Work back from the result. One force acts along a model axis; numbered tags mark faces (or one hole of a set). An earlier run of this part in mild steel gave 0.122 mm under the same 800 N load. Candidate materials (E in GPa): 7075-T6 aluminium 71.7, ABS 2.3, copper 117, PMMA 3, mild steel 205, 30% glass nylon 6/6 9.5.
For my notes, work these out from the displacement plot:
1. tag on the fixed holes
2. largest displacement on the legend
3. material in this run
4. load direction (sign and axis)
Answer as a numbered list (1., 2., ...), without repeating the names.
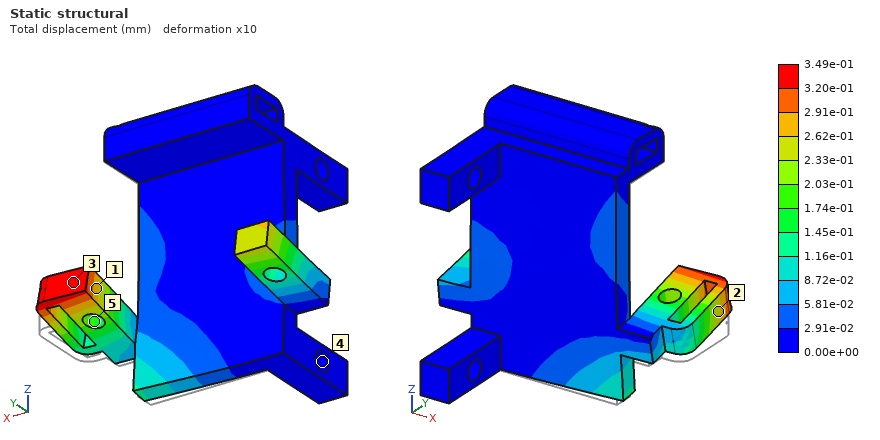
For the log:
1. 4
2. 3.49e-01 mm
3. 7075-T6 aluminium
4. +Z
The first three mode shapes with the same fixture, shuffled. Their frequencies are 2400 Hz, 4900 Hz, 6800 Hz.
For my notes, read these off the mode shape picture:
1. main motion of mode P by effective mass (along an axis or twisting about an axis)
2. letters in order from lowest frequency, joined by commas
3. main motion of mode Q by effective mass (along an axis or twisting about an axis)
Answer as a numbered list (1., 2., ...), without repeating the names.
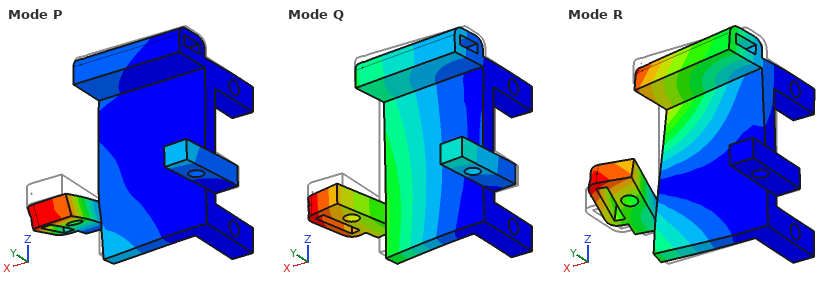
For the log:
1. along Z
2. Q, R, P
3. along Y
